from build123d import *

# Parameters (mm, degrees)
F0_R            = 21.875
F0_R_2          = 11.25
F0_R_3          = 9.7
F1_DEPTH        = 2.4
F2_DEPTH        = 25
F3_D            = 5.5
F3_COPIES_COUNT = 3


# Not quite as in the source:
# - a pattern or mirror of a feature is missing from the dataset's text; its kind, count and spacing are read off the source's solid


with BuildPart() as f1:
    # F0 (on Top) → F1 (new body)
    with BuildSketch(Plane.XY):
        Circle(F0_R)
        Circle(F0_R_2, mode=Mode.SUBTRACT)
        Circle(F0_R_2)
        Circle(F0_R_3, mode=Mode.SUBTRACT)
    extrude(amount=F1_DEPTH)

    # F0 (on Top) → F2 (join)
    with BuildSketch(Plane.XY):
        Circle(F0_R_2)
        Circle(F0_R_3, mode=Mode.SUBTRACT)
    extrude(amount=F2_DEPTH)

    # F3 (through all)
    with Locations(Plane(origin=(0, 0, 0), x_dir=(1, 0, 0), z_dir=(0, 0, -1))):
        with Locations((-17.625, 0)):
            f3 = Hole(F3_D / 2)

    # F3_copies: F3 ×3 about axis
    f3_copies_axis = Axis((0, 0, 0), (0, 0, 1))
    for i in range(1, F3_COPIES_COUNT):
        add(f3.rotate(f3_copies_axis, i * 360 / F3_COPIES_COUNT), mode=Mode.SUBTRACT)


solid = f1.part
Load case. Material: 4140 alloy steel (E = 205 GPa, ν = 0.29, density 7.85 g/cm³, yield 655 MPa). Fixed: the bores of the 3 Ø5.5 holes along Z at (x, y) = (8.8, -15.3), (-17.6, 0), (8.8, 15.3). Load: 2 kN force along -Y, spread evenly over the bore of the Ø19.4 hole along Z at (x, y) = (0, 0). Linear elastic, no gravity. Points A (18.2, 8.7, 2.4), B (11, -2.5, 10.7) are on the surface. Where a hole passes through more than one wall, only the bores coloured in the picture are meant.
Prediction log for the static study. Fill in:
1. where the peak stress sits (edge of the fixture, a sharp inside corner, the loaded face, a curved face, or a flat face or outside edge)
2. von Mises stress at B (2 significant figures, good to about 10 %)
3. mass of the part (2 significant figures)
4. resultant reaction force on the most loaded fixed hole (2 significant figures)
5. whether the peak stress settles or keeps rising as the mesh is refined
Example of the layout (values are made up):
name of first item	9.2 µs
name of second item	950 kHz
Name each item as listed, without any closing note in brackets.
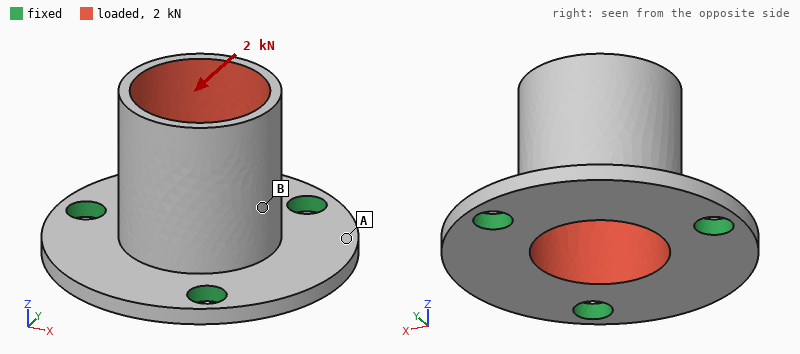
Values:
where the peak stress sits	edge of the fixture
von Mises stress at B	50 MPa
mass of the part	40 g
resultant reaction force on the most loaded fixed hole	1.1 kN
whether the peak stress settles or keeps rising as the mesh is refined	keeps rising
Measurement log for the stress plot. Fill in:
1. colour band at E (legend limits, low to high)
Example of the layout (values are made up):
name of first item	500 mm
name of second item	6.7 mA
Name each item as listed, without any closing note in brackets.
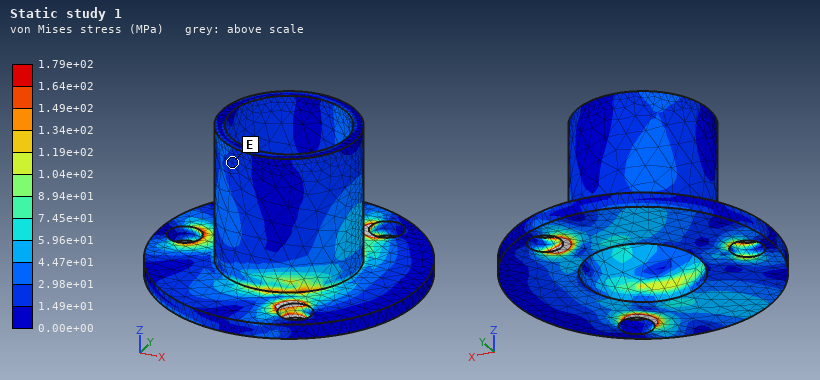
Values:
colour band at E	1.49e+01 to 2.98e+01 MPa
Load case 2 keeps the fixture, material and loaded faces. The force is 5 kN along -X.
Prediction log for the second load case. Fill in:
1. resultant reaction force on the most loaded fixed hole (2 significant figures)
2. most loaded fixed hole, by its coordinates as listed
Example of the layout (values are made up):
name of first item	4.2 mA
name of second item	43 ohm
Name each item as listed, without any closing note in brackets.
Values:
resultant reaction force on the most loaded fixed hole	3.0 kN
most loaded fixed hole, by its coordinates as listed	(-17.6, 0)
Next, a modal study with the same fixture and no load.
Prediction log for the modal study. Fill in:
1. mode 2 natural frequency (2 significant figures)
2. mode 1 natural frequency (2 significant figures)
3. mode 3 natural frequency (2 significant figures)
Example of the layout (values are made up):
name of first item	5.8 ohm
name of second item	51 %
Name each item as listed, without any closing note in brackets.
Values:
mode 2 natural frequency	8500 Hz
mode 1 natural frequency	8500 Hz
mode 3 natural frequency	12 kHz
